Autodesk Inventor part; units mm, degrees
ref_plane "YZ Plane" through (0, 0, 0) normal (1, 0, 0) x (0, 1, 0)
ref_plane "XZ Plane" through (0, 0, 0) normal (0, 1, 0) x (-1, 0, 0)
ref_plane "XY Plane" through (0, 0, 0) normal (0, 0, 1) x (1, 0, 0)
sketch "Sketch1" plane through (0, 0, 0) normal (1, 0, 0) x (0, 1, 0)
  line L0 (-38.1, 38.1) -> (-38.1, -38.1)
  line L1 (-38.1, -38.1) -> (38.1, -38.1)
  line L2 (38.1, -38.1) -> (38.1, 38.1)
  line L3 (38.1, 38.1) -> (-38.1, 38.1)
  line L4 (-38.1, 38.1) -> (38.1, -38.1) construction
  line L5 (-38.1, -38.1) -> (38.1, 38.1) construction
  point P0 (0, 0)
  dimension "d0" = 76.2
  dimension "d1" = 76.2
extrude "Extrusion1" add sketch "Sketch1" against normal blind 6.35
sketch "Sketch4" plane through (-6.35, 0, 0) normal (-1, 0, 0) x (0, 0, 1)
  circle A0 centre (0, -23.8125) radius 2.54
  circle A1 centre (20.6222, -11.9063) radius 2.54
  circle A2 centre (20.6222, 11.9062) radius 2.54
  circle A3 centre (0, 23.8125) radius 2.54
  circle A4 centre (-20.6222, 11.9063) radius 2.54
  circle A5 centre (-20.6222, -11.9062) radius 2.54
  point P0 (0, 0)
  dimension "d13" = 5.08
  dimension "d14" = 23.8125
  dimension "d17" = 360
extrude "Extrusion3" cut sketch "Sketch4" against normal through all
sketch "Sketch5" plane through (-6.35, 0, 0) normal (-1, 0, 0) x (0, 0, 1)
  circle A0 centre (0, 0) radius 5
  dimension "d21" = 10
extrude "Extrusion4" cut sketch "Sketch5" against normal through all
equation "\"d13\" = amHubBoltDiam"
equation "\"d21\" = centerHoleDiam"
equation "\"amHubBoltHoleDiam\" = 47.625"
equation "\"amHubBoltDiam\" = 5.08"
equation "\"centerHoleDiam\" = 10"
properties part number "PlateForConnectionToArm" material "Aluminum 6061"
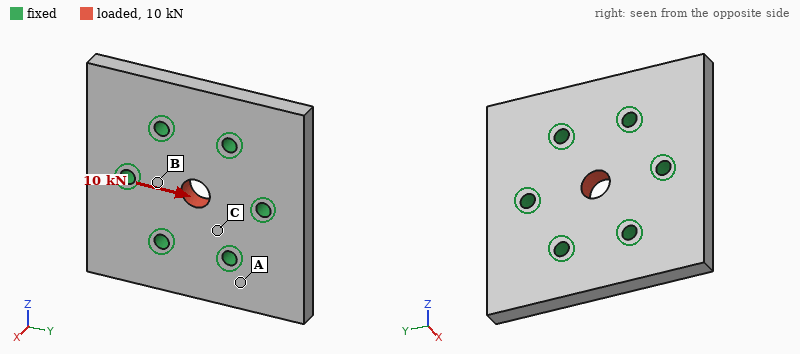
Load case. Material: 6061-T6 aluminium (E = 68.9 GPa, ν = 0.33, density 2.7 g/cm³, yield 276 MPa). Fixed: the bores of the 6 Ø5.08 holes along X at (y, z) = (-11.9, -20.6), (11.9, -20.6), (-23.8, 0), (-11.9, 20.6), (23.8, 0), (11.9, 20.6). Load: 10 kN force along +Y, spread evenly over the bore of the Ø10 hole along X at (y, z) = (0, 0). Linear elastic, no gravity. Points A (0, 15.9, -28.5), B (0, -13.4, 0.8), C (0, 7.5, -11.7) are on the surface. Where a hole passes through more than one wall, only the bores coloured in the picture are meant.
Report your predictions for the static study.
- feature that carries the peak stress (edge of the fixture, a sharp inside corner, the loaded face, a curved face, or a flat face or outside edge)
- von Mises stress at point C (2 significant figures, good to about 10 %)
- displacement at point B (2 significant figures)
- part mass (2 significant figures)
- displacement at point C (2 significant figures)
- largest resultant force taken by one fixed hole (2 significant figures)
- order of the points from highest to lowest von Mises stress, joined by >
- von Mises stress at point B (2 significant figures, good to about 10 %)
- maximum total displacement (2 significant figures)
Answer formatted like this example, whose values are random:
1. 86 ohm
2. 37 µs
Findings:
1. the loaded face
2. 20 MPa
3. 4.5 µm
4. 96 g
5. 3.1 µm
6. 2.6 kN
7. B > C > A
8. 37 MPa
9. 9.8 µm
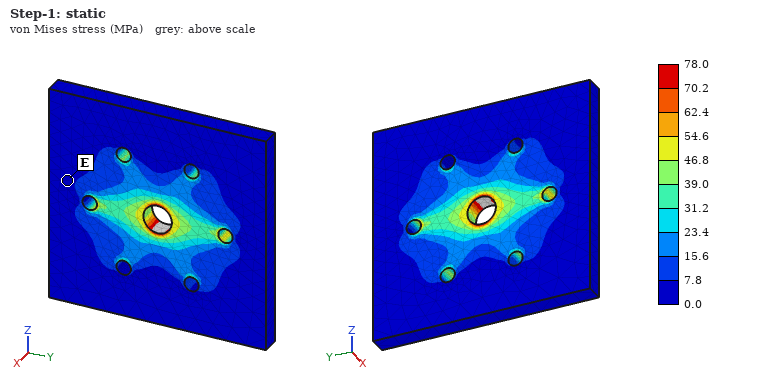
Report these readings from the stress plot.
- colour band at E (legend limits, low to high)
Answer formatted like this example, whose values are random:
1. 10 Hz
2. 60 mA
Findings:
1. 0.0 to 7.8 MPa
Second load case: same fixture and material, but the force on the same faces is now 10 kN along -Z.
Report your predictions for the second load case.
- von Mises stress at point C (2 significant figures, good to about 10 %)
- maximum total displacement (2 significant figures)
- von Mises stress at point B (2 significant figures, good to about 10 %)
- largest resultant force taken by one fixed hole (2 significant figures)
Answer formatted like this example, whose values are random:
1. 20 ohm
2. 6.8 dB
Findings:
1. 32 MPa
2. 9.9 µm
3. 9.1 MPa
4. 2.3 kN
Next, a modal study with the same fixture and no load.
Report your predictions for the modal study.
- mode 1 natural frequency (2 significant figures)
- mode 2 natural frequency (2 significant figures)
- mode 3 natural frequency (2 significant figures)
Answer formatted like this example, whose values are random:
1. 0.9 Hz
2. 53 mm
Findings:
1. 8300 Hz
2. 8400 Hz
3. 8600 Hz
